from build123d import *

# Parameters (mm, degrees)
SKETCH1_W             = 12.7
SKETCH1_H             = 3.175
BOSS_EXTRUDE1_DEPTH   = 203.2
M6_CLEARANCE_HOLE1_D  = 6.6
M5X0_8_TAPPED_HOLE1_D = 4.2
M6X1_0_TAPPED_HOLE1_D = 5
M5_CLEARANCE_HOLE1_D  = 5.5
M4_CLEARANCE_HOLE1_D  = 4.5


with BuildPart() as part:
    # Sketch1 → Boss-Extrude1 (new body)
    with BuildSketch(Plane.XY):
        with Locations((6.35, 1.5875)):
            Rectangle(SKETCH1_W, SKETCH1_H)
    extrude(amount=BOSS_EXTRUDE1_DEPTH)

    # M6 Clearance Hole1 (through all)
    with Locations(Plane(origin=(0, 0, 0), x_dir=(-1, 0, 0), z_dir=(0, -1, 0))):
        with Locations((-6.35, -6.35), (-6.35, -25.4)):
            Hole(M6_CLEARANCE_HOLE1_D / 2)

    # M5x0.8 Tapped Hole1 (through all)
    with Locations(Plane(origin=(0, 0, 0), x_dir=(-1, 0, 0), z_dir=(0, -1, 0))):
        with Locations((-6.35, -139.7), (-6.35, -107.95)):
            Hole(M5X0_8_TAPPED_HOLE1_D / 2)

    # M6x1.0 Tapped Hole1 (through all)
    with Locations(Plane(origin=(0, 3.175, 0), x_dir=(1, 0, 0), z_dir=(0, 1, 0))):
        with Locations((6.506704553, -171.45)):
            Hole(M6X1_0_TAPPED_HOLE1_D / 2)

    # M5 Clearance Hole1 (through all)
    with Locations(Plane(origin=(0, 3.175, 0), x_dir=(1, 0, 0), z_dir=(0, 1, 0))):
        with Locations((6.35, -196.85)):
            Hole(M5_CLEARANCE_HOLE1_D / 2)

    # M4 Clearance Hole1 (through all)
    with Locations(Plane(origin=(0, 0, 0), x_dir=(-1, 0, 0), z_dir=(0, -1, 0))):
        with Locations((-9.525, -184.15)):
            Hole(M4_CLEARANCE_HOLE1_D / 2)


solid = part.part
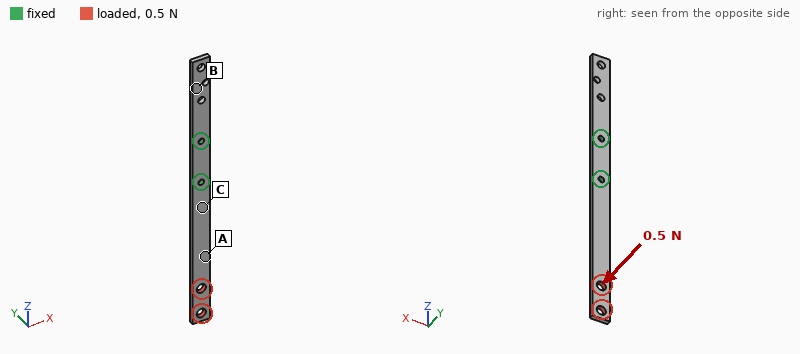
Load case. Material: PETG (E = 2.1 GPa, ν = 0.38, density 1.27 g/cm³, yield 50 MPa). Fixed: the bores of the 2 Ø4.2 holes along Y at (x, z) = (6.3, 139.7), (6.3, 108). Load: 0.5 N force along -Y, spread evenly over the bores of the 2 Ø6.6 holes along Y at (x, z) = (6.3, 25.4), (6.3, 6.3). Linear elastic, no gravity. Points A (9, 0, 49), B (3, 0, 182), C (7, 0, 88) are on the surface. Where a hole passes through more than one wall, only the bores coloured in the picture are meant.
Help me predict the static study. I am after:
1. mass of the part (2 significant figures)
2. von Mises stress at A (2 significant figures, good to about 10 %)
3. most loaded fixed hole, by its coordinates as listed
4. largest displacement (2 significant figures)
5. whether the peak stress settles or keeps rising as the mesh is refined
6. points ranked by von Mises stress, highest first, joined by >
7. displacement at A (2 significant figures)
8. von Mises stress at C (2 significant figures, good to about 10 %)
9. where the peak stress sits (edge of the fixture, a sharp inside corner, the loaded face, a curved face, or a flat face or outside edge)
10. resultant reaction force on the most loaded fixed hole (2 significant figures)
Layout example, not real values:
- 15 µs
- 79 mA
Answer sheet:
- 9.8 g
- 0.78 MPa
- (6.3, 108)
- 2.2 mm
- keeps rising
- C > A > B
- 0.84 mm
- 1.7 MPa
- edge of the fixture
- 0.51 N
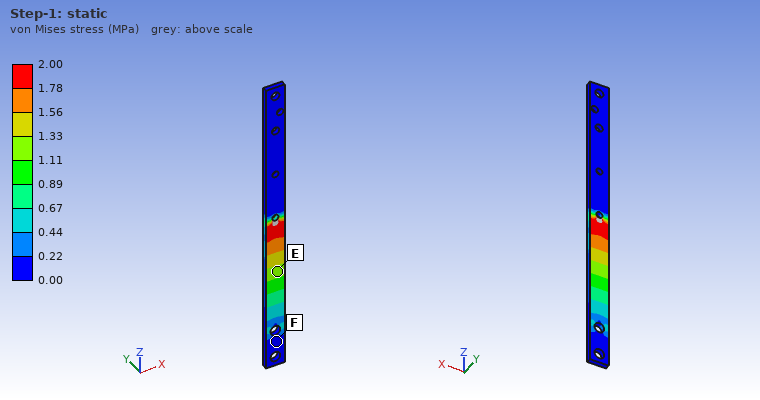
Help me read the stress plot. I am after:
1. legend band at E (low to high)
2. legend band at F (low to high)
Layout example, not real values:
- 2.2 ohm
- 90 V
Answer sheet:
- 1.11 to 1.33 MPa
- 0.00 to 0.22 MPa
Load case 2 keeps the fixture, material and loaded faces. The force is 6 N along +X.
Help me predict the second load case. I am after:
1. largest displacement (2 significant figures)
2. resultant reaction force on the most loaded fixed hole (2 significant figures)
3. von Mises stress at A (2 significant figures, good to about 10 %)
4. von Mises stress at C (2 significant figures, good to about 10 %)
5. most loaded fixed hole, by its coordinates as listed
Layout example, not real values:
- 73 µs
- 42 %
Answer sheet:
- 2.0 mm
- 14 N
- 1.0 MPa
- 0.97 MPa
- (6.3, 108)
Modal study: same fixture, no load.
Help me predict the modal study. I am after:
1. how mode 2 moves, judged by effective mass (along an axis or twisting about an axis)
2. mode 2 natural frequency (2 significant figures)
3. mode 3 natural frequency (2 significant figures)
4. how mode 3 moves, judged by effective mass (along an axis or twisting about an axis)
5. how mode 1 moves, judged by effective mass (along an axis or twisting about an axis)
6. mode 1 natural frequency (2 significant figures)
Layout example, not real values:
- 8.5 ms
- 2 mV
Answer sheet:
- along Y
- 180 Hz
- 220 Hz
- along X
- along Y
- 62 Hz
